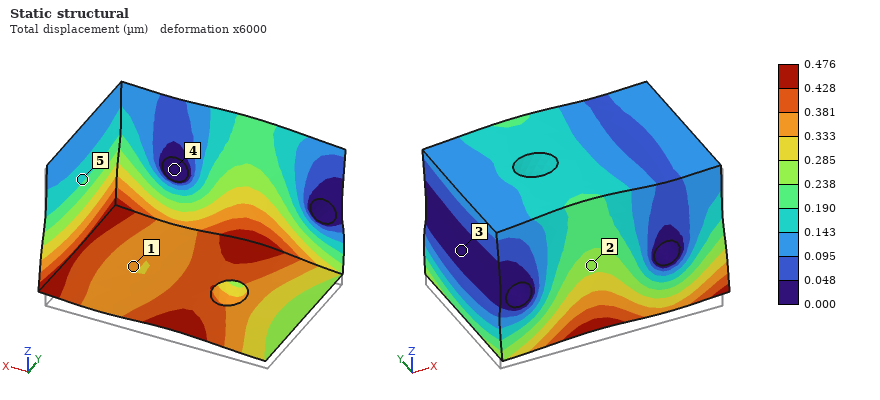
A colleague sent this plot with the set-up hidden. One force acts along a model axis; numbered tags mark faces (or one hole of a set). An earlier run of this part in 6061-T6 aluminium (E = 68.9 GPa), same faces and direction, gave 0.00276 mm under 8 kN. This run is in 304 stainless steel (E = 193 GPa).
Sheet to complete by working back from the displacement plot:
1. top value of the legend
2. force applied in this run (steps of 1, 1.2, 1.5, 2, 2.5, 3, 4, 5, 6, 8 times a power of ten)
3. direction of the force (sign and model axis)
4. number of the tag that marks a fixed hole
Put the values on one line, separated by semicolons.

0.476 µm; 4 kN; +Z; 4
